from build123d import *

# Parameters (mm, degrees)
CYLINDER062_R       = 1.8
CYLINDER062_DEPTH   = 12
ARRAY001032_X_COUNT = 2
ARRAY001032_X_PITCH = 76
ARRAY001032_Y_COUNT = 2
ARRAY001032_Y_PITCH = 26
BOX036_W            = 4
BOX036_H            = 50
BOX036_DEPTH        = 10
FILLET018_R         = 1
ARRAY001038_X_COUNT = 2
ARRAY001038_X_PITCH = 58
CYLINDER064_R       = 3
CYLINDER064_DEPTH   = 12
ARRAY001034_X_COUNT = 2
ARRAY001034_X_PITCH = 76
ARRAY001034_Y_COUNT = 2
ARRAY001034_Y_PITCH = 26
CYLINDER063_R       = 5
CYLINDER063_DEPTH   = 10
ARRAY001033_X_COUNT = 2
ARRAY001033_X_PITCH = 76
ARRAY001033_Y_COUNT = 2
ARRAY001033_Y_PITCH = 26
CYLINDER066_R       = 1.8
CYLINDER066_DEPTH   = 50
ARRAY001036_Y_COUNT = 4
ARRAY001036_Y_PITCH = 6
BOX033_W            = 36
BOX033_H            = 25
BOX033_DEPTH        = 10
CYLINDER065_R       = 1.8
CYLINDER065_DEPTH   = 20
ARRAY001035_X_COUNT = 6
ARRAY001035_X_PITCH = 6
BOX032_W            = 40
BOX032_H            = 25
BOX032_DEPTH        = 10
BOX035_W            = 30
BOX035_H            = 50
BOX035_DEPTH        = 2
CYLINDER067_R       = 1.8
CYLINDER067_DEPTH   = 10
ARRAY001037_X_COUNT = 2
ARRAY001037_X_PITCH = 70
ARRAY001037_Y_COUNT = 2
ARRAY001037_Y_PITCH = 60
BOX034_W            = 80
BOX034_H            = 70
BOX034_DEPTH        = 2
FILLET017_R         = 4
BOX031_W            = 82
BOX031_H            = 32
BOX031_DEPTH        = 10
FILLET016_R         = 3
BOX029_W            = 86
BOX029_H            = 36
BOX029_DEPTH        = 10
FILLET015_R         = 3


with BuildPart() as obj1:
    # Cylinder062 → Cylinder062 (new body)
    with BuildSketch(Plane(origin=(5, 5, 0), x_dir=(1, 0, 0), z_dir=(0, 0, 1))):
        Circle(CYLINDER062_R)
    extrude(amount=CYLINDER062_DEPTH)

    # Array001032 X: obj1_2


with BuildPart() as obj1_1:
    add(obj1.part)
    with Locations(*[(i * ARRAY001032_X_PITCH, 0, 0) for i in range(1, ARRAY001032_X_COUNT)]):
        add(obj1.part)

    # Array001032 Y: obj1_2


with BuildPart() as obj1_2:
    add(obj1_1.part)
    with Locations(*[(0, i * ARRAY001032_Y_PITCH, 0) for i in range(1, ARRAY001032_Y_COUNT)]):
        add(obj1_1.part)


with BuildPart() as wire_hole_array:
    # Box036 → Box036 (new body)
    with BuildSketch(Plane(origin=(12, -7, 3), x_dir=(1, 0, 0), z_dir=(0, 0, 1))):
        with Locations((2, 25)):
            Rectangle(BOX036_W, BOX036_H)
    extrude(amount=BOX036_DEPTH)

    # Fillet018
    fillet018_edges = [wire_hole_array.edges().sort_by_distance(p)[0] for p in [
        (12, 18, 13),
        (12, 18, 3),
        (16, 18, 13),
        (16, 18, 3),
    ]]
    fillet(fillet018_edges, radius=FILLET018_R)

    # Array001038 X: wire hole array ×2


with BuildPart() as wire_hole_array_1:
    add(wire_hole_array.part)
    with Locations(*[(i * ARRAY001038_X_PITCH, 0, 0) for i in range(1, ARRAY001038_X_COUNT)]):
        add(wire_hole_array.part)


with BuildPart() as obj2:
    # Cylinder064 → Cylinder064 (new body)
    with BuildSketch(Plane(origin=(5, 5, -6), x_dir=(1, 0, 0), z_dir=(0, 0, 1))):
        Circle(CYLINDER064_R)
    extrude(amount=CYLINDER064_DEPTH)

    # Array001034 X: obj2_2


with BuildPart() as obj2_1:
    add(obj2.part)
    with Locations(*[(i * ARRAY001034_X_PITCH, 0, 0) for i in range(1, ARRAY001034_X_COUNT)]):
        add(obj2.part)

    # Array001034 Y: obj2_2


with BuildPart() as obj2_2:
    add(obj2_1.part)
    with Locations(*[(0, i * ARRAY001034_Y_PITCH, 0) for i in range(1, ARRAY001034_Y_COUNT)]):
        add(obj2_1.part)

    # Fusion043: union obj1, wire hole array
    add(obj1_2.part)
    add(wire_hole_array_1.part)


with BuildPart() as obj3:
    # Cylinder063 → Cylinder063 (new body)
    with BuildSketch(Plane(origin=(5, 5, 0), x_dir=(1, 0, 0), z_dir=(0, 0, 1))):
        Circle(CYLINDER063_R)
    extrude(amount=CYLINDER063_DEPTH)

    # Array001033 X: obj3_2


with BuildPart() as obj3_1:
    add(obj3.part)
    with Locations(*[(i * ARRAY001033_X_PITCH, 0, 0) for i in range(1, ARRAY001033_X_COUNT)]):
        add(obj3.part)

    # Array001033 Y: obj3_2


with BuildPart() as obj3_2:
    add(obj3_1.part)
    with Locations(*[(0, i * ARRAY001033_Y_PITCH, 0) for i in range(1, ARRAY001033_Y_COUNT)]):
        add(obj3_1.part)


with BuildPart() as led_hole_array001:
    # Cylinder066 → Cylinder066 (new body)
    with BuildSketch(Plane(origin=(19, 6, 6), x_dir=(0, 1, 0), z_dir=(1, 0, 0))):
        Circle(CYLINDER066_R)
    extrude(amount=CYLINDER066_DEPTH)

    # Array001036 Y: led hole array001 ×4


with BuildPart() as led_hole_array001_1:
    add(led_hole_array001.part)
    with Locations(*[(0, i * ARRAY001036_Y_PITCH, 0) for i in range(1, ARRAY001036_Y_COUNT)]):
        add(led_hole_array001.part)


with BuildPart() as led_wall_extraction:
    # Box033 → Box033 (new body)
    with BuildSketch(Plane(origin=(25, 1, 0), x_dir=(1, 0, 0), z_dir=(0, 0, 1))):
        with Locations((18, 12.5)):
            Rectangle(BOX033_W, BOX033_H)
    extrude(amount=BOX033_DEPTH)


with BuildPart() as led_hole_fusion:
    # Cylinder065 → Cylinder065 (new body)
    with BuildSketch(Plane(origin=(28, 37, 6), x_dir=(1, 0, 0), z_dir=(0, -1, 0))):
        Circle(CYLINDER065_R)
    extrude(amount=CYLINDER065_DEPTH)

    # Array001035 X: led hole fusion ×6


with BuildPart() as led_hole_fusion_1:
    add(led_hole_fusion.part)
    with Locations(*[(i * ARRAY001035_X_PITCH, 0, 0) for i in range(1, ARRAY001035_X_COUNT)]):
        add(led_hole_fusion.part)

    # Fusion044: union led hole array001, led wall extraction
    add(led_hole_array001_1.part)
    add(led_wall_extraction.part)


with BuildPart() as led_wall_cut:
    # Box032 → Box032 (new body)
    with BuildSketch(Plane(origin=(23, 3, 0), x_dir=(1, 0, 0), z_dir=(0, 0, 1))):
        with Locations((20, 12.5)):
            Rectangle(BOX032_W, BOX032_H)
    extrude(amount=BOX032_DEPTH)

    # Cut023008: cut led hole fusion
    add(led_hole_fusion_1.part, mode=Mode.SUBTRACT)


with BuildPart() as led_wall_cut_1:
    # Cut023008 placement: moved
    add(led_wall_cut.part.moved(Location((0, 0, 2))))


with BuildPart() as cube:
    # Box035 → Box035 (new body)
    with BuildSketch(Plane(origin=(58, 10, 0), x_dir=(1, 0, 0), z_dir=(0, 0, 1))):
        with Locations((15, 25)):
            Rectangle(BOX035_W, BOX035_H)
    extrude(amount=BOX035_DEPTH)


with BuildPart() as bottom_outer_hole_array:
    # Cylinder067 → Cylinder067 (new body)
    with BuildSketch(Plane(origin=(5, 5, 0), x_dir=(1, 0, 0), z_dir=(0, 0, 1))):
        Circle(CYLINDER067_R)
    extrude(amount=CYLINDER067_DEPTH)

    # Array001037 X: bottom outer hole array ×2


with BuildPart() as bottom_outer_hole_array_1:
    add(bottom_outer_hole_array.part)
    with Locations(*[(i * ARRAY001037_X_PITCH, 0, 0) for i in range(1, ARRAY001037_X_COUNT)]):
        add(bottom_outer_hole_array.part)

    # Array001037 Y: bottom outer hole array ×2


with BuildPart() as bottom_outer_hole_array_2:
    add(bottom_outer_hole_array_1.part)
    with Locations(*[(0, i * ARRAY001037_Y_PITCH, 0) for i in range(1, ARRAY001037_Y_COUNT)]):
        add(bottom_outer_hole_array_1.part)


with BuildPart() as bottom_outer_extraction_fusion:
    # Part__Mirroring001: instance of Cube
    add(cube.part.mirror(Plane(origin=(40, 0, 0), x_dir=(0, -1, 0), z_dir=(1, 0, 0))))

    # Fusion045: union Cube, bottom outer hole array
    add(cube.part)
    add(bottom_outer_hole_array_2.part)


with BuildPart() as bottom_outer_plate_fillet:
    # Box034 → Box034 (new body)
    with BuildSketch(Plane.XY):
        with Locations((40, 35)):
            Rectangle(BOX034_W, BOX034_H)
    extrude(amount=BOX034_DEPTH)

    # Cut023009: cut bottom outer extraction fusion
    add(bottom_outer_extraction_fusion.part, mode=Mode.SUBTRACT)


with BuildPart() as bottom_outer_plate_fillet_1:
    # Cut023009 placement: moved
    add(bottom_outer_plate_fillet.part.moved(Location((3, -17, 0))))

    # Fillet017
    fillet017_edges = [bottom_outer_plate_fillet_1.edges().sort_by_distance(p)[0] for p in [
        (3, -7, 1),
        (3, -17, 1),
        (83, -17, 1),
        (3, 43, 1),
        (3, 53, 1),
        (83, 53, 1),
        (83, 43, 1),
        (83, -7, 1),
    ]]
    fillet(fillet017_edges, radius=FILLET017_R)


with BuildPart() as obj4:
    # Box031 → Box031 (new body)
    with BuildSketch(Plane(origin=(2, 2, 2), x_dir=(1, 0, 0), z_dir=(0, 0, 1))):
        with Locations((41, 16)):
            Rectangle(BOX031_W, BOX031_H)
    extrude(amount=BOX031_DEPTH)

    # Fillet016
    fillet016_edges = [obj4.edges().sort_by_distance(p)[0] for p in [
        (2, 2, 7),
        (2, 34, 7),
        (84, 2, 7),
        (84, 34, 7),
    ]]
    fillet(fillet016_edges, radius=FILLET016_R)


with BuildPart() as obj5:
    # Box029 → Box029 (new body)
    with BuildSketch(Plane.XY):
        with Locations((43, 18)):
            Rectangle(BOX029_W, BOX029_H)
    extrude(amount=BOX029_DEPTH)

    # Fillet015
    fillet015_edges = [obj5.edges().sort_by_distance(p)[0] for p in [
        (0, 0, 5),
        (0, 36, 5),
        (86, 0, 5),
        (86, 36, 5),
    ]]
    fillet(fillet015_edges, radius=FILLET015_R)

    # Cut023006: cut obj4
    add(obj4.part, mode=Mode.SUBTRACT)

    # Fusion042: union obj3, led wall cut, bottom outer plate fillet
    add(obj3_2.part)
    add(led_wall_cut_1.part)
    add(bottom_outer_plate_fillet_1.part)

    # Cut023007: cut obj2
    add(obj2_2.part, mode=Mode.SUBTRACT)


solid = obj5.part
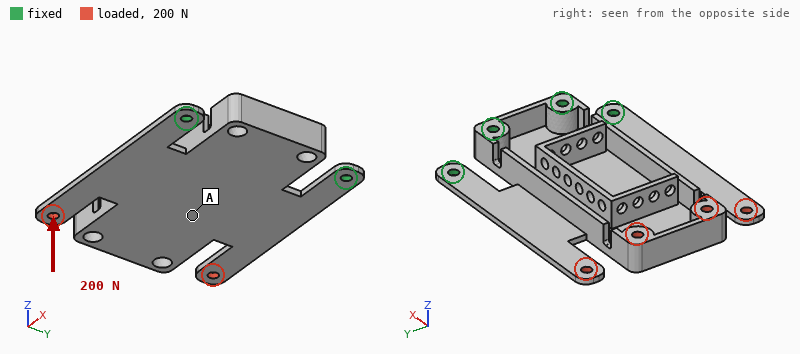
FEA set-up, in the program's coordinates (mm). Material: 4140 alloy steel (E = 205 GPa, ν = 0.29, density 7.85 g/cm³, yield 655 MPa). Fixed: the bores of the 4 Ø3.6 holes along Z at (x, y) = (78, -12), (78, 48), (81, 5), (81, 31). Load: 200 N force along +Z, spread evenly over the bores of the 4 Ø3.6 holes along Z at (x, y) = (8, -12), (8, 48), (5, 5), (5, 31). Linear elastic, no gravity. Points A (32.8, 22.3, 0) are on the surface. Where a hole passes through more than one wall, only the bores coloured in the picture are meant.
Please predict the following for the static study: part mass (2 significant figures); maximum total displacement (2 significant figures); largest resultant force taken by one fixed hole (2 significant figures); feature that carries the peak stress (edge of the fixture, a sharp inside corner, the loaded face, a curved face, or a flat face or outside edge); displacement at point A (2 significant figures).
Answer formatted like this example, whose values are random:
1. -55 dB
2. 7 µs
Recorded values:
1. 130 g
2. 1.3 mm
3. 490 N
4. a curved face
5. 0.61 mm
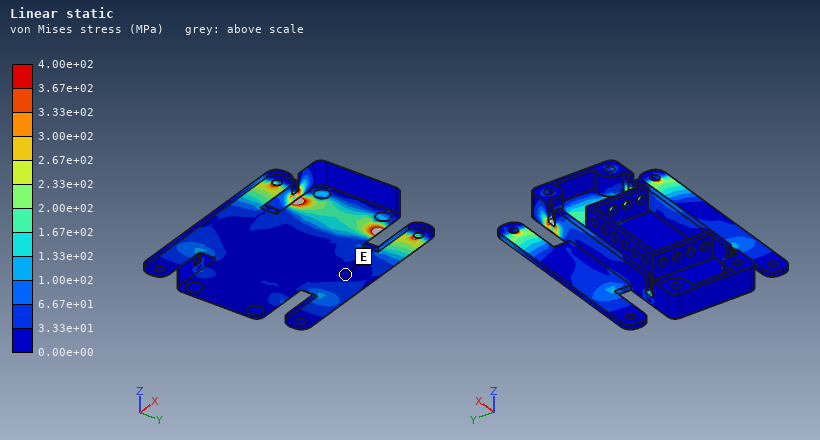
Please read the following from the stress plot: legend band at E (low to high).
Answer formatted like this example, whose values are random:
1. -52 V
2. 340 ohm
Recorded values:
1. 0.00e+00 to 3.33e+01 MPa
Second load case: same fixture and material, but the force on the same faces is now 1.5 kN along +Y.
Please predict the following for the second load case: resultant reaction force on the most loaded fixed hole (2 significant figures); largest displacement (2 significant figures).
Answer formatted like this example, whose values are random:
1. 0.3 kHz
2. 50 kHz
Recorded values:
1. 1.6 kN
2. 0.56 mm
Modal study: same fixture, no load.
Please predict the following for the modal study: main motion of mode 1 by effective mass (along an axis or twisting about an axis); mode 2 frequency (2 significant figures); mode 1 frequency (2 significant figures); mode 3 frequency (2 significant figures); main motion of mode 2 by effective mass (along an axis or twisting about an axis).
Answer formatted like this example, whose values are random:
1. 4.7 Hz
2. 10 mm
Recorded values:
1. along Z
2. 840 Hz
3. 340 Hz
4. 1900 Hz
5. twisting about X
